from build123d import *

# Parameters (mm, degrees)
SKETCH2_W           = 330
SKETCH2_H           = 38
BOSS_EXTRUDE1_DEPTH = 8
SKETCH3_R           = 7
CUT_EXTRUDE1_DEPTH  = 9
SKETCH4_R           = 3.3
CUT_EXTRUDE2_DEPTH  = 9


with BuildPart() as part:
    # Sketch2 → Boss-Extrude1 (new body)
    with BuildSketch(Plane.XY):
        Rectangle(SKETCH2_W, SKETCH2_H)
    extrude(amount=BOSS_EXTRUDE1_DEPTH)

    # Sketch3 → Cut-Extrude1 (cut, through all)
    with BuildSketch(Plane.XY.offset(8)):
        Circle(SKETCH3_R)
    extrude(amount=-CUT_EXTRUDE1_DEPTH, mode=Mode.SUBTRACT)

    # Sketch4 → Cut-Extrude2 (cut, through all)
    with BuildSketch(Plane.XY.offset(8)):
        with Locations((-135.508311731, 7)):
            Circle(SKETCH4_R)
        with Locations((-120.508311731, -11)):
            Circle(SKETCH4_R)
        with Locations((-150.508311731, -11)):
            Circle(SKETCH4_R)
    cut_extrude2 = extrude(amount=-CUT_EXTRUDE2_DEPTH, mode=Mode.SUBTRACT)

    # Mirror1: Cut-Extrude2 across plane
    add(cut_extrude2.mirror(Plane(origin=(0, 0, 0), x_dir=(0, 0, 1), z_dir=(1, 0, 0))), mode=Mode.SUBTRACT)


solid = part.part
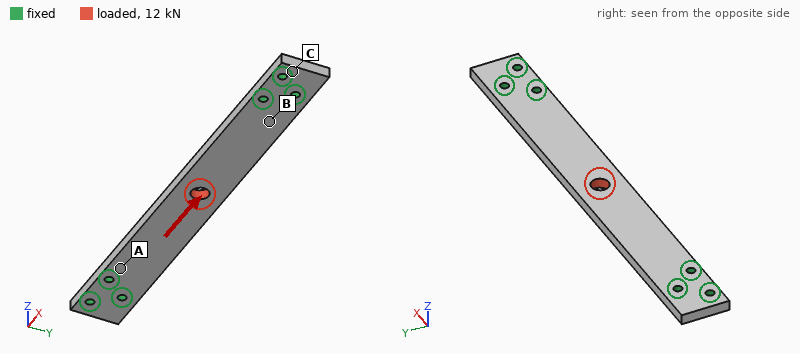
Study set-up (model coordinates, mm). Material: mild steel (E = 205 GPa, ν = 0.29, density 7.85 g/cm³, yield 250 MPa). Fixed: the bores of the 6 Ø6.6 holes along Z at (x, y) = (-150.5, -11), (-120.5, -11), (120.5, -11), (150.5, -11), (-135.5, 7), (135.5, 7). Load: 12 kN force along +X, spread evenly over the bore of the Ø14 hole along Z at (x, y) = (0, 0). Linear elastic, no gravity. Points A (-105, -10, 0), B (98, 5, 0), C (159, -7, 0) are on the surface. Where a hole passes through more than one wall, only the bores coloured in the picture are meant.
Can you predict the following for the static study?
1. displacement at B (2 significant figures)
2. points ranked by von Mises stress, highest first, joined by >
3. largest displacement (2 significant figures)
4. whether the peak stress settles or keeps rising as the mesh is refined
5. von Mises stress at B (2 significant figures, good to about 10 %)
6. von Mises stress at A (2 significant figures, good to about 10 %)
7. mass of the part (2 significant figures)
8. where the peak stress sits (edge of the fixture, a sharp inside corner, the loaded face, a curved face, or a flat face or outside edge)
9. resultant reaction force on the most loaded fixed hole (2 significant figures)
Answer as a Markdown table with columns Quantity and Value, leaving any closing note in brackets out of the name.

| Quantity | Value |
|---|---|
| displacement at B | 3.2 µm |
| points ranked by von Mises stress, highest first, joined by > | A > B > C |
| largest displacement | 13 µm |
| whether the peak stress settles or keeps rising as the mesh is refined | keeps rising |
| von Mises stress at B | 18 MPa |
| von Mises stress at A | 24 MPa |
| mass of the part | 760 g |
| where the peak stress sits | edge of the fixture |
| resultant reaction force on the most loaded fixed hole | 3.3 kN |
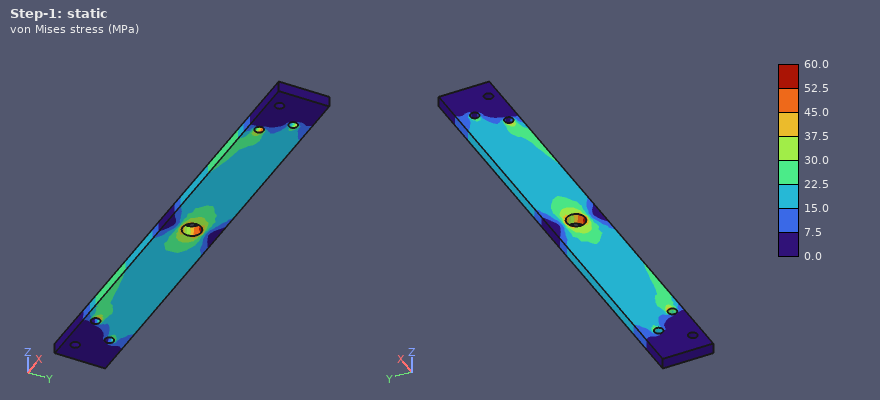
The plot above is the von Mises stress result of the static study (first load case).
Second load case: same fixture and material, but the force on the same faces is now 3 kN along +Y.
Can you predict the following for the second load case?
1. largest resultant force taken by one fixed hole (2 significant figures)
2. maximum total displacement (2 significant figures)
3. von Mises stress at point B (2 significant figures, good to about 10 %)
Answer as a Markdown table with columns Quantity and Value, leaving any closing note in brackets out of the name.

| Quantity | Value |
|---|---|
| largest resultant force taken by one fixed hole | 3.9 kN |
| maximum total displacement | 43 µm |
| von Mises stress at point B | 13 MPa |
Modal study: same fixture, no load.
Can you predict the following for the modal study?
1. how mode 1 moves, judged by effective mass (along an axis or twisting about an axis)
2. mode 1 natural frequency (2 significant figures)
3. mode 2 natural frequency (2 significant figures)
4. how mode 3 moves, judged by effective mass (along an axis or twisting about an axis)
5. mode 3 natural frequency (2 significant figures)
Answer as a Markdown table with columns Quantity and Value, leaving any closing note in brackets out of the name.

| Quantity | Value |
|---|---|
| how mode 1 moves, judged by effective mass | along Z |
| mode 1 natural frequency | 690 Hz |
| mode 2 natural frequency | 1900 Hz |
| how mode 3 moves, judged by effective mass | twisting about X |
| mode 3 natural frequency | 2600 Hz |
